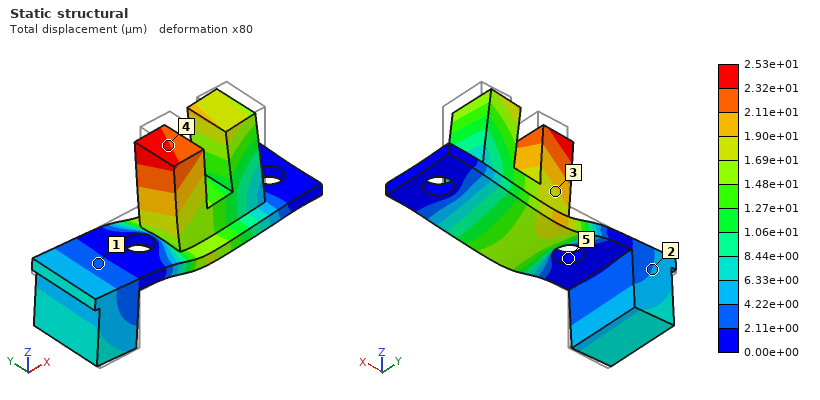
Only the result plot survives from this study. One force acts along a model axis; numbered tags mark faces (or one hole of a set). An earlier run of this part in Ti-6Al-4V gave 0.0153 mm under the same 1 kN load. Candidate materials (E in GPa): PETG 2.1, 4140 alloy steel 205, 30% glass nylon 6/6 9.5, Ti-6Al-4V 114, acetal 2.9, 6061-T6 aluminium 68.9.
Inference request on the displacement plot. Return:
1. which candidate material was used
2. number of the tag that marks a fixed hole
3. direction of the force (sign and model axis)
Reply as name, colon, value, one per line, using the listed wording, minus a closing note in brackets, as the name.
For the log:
which candidate material was used: 6061-T6 aluminium
number of the tag that marks a fixed hole: 5
direction of the force: -Z
